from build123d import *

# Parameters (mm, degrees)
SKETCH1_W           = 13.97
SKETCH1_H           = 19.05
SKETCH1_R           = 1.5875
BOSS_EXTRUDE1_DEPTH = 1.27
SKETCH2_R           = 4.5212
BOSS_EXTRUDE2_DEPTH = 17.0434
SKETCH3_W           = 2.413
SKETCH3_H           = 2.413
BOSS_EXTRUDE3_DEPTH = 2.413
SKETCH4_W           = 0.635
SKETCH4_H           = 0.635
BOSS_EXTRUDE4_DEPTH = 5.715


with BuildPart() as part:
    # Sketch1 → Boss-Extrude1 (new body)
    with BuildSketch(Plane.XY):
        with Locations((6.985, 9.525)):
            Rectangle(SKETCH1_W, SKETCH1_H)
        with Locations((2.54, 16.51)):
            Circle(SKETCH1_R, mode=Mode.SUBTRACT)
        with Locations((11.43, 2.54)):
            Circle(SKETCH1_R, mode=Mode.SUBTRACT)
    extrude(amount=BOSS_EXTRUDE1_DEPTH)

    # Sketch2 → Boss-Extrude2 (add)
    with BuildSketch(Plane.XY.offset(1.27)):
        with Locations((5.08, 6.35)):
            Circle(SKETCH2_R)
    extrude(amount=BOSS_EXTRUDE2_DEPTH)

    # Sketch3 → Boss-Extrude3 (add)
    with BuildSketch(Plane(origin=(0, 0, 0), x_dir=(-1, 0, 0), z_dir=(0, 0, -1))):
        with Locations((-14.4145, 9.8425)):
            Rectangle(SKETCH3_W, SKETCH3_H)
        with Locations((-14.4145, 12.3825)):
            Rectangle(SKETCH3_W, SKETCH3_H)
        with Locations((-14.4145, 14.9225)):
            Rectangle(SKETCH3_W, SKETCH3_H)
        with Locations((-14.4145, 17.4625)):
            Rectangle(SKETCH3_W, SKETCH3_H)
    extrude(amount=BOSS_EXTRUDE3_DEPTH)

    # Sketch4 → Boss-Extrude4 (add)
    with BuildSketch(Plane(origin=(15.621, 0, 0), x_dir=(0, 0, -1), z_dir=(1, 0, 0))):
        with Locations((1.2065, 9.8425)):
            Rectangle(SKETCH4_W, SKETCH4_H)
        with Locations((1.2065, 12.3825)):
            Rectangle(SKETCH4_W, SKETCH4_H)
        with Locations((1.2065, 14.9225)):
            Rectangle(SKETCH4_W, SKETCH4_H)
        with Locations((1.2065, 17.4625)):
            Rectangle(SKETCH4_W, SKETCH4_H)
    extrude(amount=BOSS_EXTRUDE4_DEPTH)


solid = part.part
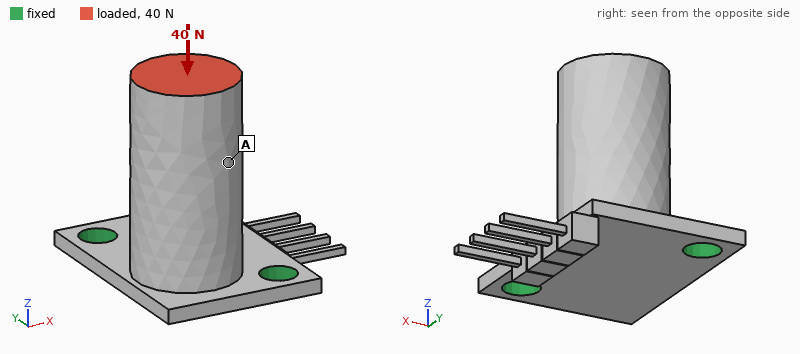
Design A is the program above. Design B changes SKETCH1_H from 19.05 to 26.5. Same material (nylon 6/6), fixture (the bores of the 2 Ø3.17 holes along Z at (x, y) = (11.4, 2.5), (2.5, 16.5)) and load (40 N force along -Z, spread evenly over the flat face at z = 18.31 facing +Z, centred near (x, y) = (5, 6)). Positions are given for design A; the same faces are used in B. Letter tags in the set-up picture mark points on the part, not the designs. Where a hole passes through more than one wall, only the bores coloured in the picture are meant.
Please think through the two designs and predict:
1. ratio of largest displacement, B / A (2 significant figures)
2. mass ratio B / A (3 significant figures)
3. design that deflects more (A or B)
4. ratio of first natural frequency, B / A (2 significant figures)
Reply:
0.88
1.09
A
1.1
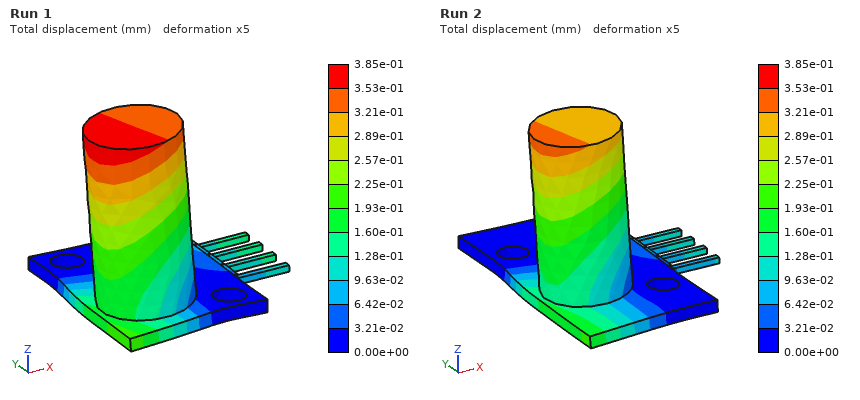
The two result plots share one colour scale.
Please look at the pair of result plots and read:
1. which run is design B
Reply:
Run 2
